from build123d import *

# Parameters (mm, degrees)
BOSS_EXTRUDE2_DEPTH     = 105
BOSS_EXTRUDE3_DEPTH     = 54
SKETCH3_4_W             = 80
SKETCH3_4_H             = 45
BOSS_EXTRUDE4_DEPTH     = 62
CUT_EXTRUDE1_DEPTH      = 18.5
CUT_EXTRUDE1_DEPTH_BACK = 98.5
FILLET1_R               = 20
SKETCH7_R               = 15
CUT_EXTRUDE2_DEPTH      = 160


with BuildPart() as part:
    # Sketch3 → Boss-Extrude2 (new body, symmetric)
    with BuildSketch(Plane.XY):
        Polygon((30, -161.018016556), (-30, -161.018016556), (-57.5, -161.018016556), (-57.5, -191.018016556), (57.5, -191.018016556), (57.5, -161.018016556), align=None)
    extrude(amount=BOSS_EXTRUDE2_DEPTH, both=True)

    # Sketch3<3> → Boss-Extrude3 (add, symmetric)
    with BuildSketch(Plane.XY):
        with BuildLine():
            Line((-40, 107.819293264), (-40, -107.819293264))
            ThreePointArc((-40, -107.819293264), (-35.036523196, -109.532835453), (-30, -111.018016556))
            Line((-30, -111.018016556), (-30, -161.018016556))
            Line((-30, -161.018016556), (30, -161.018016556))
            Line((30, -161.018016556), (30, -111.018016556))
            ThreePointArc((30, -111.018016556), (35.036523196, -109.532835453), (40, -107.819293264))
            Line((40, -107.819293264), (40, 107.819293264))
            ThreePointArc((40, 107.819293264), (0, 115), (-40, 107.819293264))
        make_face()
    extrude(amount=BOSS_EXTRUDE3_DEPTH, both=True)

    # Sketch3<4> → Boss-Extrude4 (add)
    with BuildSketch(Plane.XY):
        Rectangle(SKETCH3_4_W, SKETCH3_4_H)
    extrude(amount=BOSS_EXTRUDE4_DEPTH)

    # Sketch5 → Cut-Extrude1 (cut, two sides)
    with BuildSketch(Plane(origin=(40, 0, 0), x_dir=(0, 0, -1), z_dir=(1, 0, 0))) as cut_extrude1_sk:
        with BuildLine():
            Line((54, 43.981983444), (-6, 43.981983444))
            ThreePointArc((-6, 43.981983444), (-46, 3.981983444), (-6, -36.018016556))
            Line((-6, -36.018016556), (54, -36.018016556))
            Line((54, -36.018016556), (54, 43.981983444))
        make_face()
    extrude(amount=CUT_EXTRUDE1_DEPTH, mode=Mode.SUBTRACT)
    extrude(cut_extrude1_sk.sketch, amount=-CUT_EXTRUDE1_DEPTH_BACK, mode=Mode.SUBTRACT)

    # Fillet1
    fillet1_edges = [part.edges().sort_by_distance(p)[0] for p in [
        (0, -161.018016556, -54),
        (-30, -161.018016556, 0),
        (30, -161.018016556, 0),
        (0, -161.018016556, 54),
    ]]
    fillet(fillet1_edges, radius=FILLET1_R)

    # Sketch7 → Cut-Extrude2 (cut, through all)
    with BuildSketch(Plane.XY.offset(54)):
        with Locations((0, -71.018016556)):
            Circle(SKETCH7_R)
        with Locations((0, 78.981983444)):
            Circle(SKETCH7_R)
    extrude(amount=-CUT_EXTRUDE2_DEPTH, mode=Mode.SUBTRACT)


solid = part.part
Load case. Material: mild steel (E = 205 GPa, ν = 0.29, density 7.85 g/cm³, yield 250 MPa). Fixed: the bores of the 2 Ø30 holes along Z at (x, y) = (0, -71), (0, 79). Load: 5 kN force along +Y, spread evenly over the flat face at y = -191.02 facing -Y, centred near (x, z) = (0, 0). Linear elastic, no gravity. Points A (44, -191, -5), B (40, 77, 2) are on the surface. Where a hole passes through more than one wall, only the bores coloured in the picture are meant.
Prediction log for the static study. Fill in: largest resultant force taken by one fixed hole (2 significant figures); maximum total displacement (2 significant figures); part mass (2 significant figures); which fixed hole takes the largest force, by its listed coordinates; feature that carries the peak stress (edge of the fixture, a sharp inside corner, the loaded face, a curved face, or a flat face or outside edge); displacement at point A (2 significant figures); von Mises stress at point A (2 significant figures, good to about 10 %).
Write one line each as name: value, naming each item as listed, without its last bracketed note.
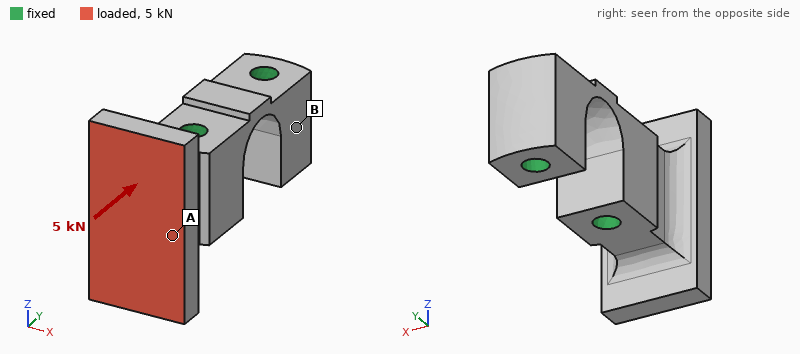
largest resultant force taken by one fixed hole: 5.0 kN
maximum total displacement: 1.5 µm
part mass: 18 kg
which fixed hole takes the largest force, by its listed coordinates: (0, -71)
feature that carries the peak stress: a curved face
displacement at point A: 0.27 µm
von Mises stress at point A: 0.93 MPa
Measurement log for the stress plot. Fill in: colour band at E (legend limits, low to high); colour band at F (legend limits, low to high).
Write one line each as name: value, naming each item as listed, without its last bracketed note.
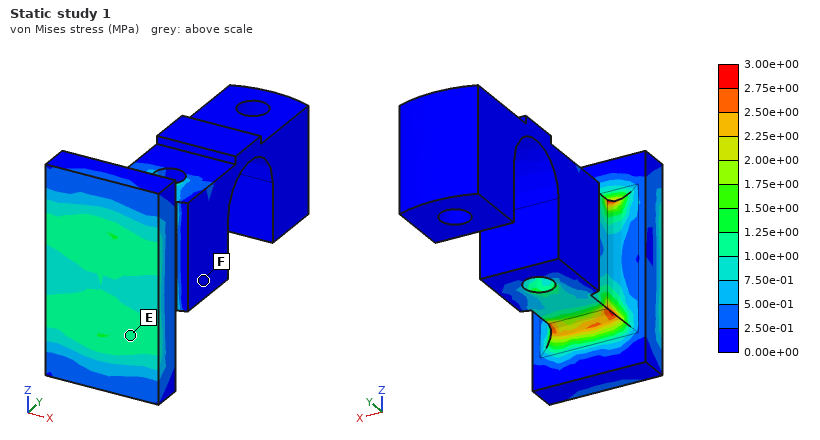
colour band at E: 1.00e+00 to 1.25e+00 MPa
colour band at F: 0.00e+00 to 2.50e-01 MPa
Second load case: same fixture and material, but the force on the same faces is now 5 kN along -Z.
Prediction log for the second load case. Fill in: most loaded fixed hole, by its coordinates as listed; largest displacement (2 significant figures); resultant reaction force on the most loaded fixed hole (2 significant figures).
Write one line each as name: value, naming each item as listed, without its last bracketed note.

most loaded fixed hole, by its coordinates as listed: (0, -71)
largest displacement: 4.5 µm
resultant reaction force on the most loaded fixed hole: 5.0 kN
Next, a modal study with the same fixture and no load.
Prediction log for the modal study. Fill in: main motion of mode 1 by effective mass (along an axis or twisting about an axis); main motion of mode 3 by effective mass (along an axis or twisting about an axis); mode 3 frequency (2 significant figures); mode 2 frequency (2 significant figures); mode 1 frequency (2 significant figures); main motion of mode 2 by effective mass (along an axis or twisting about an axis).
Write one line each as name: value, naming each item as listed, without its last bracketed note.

main motion of mode 1 by effective mass: along X
main motion of mode 3 by effective mass: along Z
mode 3 frequency: 2500 Hz
mode 2 frequency: 2300 Hz
mode 1 frequency: 1800 Hz
main motion of mode 2 by effective mass: twisting about Y
